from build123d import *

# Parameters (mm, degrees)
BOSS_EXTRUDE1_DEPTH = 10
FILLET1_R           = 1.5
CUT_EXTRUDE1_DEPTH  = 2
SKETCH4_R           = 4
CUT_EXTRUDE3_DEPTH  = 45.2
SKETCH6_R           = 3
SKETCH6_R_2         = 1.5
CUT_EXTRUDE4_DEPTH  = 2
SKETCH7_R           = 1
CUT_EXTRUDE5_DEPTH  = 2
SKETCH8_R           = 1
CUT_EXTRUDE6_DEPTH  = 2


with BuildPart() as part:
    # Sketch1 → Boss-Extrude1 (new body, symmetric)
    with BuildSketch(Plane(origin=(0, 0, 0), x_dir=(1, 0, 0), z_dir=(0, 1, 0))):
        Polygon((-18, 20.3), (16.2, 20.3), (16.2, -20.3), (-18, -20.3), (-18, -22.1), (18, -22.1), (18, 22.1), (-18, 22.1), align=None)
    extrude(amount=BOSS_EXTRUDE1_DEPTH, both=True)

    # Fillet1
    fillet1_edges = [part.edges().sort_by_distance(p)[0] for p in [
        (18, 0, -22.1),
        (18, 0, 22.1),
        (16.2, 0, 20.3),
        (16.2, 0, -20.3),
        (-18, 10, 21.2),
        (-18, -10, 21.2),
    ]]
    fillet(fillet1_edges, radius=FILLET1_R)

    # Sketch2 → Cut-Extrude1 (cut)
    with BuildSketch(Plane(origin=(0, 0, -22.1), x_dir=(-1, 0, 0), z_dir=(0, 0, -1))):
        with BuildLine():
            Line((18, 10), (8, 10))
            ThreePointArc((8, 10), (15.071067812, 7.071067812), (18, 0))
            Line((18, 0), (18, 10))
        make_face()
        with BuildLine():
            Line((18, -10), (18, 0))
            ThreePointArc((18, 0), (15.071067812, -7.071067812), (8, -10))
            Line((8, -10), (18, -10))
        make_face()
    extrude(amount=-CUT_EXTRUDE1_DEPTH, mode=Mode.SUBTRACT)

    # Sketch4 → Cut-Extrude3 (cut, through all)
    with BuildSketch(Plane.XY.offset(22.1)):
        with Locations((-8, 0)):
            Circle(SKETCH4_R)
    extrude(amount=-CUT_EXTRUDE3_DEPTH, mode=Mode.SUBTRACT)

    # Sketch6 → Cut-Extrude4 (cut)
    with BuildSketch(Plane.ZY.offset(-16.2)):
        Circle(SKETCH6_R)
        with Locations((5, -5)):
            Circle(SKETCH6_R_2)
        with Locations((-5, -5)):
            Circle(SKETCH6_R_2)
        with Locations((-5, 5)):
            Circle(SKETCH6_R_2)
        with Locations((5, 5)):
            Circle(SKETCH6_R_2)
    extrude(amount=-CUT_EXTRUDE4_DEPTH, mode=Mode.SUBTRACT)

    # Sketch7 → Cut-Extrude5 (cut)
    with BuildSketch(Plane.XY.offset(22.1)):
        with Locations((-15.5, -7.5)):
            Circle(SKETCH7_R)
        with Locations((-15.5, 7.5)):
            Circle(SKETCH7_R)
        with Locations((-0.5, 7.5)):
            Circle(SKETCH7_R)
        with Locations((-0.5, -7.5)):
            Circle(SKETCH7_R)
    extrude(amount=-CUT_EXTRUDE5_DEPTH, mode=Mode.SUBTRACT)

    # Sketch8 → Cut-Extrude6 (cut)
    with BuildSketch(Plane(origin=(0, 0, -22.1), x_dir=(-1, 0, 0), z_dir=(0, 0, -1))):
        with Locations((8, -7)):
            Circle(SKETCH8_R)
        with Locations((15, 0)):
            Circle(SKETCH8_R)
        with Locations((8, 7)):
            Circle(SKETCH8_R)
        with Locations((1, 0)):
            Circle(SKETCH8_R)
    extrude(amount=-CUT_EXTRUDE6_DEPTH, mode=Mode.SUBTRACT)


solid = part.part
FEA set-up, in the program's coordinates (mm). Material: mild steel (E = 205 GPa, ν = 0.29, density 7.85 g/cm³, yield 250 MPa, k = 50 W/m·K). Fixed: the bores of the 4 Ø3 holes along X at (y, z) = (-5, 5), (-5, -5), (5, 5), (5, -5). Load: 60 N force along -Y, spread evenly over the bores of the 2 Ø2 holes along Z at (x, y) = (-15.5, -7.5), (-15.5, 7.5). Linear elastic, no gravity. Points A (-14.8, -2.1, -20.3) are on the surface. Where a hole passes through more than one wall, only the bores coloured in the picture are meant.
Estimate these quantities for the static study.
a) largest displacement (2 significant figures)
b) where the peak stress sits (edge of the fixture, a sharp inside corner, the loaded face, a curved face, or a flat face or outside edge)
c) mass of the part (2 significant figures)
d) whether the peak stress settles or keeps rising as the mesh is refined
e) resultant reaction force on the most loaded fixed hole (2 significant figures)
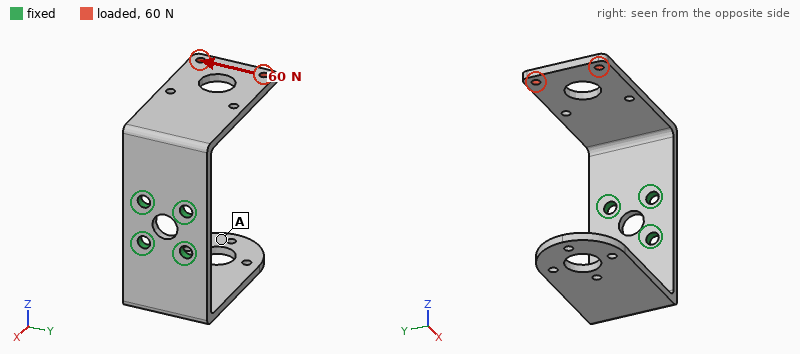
0.21 mm
edge of the fixture
29 g
keeps rising
170 N
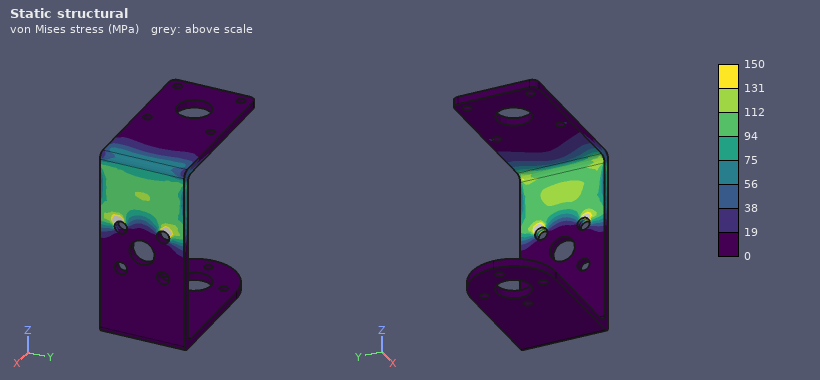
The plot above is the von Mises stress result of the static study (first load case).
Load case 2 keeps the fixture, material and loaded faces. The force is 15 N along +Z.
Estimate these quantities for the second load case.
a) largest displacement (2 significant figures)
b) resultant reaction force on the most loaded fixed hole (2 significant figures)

0.21 mm
7.8 N
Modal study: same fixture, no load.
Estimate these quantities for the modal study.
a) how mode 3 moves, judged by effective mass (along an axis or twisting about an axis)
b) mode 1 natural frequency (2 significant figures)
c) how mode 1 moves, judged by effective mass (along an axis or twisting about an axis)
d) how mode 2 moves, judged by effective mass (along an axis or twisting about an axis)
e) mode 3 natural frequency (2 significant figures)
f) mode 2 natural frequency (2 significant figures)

along Y
790 Hz
along Z
along Z
1500 Hz
880 Hz
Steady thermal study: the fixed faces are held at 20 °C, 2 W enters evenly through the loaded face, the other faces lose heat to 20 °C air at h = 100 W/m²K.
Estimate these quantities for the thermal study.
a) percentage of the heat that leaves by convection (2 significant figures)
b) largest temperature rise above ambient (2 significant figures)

84 %
25 K
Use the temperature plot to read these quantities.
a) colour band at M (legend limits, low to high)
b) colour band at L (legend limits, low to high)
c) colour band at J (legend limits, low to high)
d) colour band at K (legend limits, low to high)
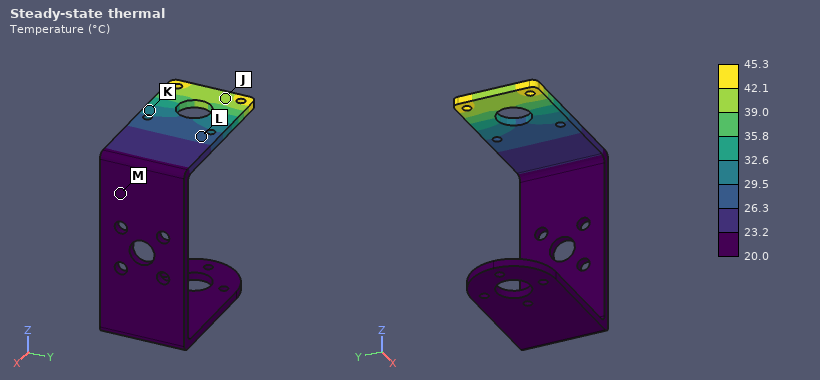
20.0 to 23.2 °C
26.3 to 29.5 °C
39.0 to 42.1 °C
29.5 to 32.6 °C
